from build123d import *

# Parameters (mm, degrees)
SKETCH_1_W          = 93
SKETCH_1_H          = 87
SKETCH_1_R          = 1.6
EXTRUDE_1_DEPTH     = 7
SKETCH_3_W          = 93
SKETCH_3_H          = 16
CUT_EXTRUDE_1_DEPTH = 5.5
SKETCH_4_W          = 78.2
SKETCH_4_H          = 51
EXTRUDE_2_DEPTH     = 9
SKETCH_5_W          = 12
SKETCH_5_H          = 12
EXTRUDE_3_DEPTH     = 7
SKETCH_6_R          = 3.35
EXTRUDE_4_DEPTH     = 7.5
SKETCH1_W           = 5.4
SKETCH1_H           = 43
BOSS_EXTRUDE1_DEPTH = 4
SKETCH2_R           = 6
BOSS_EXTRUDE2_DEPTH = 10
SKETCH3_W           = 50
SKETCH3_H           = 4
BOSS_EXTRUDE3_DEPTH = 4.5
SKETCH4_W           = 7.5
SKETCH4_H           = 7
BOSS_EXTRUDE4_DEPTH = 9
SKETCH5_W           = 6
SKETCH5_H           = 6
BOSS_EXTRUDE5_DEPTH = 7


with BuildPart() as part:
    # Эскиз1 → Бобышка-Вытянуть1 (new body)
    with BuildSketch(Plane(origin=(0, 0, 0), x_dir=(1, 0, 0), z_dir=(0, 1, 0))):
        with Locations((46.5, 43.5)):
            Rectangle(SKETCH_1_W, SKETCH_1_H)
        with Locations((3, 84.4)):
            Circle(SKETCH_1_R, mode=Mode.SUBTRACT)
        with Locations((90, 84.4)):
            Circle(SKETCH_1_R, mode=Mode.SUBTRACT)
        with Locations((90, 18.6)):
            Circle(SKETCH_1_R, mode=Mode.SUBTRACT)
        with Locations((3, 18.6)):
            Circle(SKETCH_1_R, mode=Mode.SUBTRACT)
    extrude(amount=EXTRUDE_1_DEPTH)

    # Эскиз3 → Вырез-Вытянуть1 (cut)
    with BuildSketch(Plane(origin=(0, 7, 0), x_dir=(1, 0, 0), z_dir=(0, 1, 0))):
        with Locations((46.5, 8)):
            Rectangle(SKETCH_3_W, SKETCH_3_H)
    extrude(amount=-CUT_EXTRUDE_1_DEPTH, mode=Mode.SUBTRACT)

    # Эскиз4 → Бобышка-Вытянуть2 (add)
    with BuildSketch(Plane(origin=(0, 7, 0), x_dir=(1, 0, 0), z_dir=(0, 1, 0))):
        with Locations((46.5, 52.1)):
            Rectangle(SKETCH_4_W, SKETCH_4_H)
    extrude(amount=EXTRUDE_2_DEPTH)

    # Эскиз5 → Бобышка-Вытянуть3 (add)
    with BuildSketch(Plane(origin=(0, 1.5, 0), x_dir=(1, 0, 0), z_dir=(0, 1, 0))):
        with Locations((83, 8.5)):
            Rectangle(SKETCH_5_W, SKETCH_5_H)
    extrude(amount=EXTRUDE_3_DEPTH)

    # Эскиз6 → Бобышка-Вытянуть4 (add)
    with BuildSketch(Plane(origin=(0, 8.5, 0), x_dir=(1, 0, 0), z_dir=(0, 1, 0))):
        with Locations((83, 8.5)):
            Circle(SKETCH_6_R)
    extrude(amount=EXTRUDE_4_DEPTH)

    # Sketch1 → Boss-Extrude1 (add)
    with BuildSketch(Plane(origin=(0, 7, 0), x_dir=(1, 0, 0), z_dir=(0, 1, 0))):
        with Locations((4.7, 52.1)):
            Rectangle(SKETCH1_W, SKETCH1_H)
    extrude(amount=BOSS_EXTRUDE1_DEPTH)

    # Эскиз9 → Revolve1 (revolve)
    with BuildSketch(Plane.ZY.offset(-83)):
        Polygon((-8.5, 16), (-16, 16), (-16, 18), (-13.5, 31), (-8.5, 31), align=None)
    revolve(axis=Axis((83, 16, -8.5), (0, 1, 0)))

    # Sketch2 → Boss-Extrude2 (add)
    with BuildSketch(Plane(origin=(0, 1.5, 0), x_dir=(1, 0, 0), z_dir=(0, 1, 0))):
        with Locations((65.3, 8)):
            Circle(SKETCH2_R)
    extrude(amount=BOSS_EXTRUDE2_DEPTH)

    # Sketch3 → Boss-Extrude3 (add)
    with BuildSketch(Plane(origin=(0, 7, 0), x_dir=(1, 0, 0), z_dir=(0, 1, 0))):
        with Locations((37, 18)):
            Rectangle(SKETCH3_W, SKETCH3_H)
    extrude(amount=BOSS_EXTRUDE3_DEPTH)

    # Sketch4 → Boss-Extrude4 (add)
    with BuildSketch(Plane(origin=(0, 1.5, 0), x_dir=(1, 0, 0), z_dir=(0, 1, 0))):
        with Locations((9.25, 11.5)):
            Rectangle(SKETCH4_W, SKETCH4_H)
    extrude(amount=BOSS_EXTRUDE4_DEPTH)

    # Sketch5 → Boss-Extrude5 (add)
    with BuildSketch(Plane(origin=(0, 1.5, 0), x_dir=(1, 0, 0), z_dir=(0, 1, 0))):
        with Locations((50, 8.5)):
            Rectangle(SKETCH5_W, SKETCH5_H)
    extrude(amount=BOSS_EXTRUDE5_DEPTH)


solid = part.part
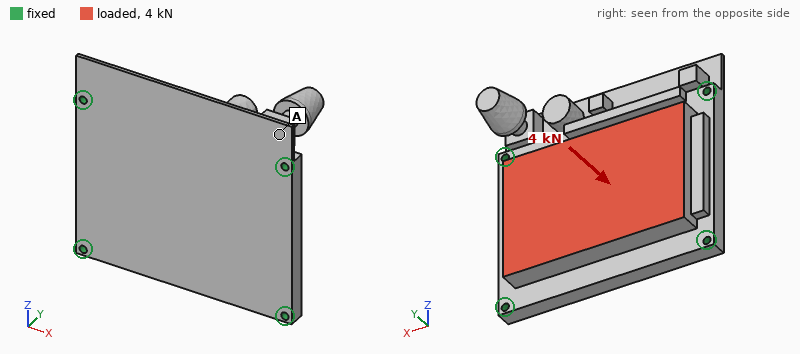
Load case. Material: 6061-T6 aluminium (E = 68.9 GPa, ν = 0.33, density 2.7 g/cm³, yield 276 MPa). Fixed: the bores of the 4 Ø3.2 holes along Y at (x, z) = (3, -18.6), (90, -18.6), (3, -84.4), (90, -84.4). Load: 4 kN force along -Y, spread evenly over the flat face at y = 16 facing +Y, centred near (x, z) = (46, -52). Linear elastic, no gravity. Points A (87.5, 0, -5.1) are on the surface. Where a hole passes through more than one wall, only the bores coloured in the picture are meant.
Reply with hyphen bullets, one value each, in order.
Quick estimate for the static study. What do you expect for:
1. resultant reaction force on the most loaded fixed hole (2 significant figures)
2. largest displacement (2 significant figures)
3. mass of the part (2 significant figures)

- 1.3 kN
- 32 µm
- 250 g
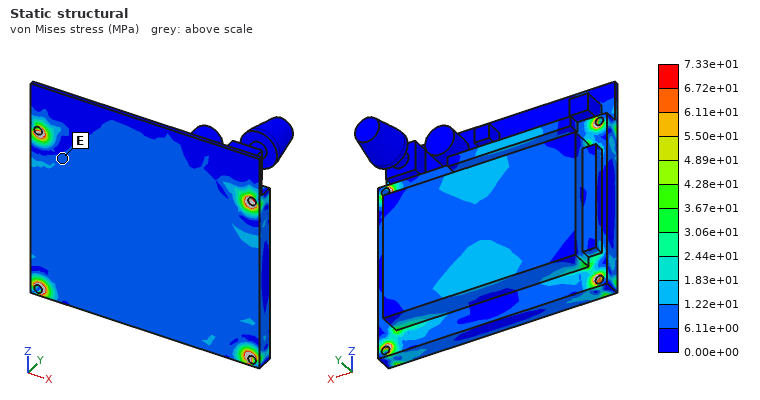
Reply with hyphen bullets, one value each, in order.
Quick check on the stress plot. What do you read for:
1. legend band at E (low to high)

- 6.11e+00 to 1.22e+01 MPa
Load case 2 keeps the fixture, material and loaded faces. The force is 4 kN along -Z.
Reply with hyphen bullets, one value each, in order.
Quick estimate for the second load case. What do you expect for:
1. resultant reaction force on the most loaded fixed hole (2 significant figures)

- 1.2 kN
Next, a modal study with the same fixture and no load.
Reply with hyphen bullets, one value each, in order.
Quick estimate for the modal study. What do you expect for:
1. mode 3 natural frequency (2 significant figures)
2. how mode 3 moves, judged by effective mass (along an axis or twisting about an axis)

- 4100 Hz
- along Y
